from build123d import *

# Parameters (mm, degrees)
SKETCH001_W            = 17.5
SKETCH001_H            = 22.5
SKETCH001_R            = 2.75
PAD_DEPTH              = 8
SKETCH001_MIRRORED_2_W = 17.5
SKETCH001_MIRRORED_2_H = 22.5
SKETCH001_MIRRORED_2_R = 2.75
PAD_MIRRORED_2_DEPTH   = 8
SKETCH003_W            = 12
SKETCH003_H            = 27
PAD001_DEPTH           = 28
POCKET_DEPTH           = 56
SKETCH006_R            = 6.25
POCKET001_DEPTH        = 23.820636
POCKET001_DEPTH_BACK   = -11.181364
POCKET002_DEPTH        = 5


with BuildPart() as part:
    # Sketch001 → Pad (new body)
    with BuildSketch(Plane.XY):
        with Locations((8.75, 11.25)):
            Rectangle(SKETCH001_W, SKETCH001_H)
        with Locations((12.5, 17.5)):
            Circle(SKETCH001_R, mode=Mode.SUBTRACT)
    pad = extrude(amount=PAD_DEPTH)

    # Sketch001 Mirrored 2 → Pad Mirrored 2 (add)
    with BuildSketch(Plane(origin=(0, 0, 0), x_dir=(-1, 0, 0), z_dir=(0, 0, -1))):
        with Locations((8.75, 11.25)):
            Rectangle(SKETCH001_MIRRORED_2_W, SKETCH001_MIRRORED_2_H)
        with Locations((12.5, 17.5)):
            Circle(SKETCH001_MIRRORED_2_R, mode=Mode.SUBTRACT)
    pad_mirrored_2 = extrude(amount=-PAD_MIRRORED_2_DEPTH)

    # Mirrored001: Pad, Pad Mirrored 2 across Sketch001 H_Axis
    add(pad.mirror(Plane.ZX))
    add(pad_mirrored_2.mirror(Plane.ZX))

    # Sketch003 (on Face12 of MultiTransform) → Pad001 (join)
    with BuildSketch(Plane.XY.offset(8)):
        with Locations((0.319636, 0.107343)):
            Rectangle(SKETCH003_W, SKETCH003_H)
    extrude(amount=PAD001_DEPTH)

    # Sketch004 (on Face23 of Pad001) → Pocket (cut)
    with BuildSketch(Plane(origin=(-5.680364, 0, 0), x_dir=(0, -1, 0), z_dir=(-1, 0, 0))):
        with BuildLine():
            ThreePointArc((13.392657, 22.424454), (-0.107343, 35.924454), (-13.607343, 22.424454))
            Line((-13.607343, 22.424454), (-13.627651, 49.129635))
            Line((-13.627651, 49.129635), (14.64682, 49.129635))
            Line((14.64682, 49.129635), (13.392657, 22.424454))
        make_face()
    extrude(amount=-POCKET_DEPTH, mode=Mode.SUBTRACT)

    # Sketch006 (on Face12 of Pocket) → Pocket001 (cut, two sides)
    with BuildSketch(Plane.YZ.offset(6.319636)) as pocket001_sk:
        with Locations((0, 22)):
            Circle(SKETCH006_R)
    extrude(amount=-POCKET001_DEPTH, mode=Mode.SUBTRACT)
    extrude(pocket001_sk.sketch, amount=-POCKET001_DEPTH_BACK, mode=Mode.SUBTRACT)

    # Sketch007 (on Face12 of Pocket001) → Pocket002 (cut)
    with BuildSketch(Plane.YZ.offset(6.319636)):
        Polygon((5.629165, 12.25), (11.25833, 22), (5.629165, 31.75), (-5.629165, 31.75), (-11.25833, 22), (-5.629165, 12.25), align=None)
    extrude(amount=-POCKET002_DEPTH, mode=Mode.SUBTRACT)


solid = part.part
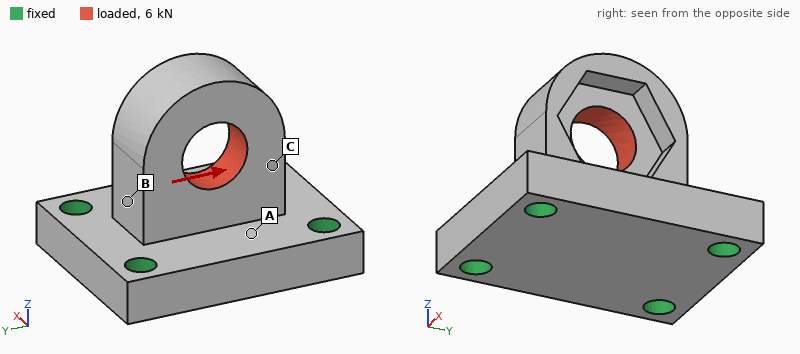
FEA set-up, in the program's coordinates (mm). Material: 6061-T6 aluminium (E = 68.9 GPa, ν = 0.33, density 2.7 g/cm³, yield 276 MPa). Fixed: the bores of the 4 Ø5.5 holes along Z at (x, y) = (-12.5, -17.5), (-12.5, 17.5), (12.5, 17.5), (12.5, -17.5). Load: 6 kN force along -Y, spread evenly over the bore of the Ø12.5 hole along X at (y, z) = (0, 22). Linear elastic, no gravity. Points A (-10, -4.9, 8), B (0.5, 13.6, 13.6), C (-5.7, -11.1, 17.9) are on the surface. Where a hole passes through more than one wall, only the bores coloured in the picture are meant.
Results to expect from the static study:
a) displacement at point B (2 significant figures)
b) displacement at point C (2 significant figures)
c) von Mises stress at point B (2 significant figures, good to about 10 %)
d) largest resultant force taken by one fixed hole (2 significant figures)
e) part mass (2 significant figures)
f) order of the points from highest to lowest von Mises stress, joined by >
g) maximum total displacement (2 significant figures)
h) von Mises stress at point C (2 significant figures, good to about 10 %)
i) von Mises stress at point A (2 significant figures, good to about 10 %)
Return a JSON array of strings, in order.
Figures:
["26 µm", "37 µm", "85 MPa", "2.5 kN", "47 g", "B > C > A", "85 µm", "60 MPa", "28 MPa"]
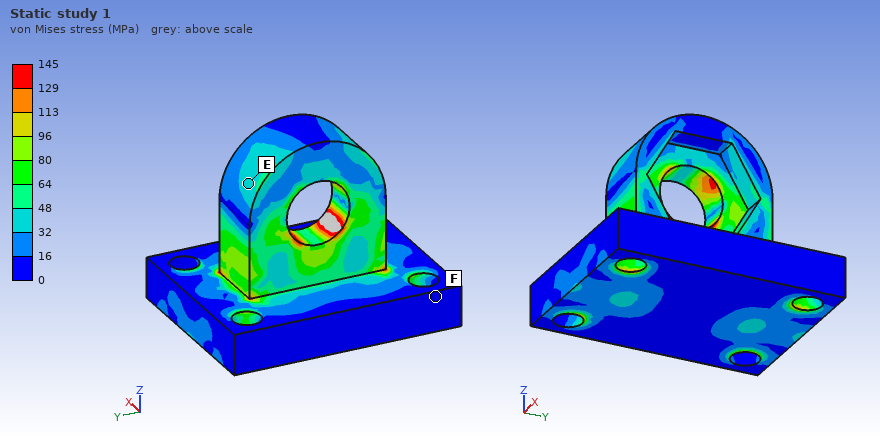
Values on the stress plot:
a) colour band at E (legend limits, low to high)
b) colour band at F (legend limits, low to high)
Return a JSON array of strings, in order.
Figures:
["32 to 48 MPa", "0 to 16 MPa"]
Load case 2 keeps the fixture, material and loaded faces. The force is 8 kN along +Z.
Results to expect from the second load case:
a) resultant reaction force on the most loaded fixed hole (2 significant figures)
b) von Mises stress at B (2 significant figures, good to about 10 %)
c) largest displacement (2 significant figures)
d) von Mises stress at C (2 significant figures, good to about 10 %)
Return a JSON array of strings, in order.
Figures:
["2.5 kN", "36 MPa", "53 µm", "56 MPa"]
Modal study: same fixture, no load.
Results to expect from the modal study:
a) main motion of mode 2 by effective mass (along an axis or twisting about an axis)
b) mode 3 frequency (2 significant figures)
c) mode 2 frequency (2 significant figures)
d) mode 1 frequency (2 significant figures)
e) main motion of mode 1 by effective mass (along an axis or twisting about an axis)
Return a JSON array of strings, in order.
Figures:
["along Y", "19 kHz", "13 kHz", "9000 Hz", "along X"]
